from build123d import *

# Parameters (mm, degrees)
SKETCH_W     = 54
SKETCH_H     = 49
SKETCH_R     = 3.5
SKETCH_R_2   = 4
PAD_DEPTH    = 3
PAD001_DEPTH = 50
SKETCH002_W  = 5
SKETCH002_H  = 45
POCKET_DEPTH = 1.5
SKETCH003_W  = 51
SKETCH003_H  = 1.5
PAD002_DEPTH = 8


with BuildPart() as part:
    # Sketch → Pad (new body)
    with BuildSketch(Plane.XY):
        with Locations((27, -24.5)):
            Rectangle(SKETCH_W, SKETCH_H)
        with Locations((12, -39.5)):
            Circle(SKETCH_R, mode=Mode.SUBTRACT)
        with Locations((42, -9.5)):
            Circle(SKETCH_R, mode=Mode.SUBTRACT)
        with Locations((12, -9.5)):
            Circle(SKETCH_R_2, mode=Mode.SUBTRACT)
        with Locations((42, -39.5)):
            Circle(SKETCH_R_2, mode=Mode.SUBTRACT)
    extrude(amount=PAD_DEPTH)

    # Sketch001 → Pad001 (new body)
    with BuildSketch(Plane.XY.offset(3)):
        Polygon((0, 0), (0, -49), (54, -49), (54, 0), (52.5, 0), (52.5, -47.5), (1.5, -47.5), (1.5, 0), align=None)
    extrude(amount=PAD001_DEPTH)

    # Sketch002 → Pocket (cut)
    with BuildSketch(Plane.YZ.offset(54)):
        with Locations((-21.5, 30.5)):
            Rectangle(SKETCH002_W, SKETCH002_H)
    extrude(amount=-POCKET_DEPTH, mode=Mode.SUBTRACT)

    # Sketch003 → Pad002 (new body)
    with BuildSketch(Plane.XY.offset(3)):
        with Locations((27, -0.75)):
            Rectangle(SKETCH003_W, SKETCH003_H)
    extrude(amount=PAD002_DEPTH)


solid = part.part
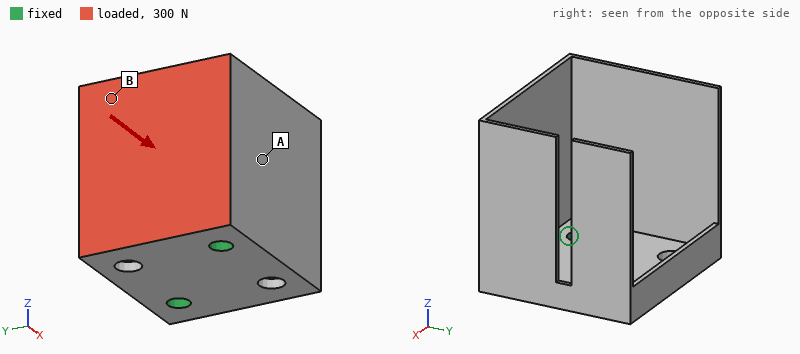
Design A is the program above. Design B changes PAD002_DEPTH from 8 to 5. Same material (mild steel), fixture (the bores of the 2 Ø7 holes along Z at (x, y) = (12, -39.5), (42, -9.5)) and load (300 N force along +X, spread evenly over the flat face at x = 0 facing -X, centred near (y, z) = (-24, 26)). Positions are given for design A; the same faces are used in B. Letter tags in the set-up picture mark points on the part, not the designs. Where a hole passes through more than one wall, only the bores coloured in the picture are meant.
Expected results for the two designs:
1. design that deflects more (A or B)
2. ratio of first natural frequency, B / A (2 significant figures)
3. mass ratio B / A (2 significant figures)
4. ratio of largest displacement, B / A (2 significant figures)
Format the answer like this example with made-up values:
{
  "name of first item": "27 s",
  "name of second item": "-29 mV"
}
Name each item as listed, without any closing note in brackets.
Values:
{
  "design that deflects more": "B",
  "ratio of first natural frequency, B / A": "0.92",
  "mass ratio B / A": "0.99",
  "ratio of largest displacement, B / A": "1.1"
}
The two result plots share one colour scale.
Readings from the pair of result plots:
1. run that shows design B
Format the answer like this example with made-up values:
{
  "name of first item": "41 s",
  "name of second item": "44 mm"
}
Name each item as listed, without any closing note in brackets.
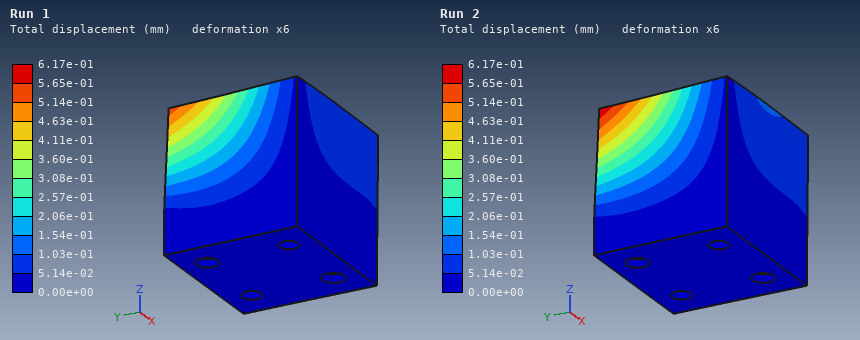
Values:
{
  "run that shows design B": "Run 2"
}
